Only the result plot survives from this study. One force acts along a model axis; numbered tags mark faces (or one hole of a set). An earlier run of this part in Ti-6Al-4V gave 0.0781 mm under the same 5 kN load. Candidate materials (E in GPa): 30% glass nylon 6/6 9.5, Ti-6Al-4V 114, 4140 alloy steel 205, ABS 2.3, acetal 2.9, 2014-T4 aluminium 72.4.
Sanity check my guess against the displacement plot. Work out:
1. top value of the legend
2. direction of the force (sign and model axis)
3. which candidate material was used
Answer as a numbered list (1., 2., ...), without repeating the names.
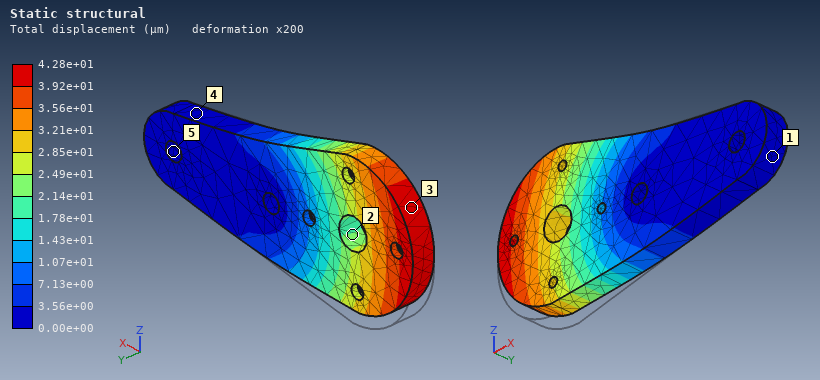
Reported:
1. 4.28e+01 µm
2. +Z
3. 4140 alloy steel
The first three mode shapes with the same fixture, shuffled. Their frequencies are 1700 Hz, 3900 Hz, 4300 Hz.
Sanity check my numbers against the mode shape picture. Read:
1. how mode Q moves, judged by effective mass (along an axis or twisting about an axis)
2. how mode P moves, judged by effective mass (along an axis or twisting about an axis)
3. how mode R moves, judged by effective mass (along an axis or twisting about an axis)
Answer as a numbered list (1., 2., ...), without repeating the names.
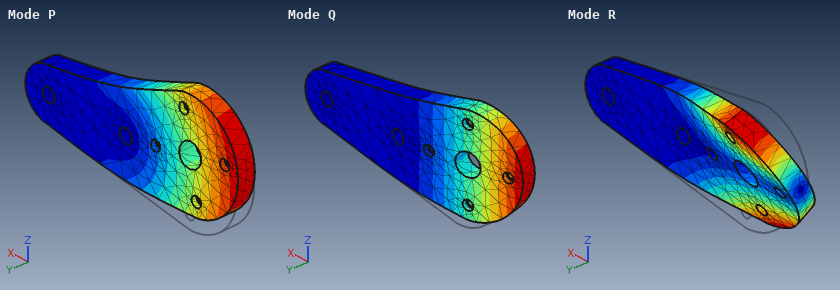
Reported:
1. along Y
2. along Z
3. twisting about X
